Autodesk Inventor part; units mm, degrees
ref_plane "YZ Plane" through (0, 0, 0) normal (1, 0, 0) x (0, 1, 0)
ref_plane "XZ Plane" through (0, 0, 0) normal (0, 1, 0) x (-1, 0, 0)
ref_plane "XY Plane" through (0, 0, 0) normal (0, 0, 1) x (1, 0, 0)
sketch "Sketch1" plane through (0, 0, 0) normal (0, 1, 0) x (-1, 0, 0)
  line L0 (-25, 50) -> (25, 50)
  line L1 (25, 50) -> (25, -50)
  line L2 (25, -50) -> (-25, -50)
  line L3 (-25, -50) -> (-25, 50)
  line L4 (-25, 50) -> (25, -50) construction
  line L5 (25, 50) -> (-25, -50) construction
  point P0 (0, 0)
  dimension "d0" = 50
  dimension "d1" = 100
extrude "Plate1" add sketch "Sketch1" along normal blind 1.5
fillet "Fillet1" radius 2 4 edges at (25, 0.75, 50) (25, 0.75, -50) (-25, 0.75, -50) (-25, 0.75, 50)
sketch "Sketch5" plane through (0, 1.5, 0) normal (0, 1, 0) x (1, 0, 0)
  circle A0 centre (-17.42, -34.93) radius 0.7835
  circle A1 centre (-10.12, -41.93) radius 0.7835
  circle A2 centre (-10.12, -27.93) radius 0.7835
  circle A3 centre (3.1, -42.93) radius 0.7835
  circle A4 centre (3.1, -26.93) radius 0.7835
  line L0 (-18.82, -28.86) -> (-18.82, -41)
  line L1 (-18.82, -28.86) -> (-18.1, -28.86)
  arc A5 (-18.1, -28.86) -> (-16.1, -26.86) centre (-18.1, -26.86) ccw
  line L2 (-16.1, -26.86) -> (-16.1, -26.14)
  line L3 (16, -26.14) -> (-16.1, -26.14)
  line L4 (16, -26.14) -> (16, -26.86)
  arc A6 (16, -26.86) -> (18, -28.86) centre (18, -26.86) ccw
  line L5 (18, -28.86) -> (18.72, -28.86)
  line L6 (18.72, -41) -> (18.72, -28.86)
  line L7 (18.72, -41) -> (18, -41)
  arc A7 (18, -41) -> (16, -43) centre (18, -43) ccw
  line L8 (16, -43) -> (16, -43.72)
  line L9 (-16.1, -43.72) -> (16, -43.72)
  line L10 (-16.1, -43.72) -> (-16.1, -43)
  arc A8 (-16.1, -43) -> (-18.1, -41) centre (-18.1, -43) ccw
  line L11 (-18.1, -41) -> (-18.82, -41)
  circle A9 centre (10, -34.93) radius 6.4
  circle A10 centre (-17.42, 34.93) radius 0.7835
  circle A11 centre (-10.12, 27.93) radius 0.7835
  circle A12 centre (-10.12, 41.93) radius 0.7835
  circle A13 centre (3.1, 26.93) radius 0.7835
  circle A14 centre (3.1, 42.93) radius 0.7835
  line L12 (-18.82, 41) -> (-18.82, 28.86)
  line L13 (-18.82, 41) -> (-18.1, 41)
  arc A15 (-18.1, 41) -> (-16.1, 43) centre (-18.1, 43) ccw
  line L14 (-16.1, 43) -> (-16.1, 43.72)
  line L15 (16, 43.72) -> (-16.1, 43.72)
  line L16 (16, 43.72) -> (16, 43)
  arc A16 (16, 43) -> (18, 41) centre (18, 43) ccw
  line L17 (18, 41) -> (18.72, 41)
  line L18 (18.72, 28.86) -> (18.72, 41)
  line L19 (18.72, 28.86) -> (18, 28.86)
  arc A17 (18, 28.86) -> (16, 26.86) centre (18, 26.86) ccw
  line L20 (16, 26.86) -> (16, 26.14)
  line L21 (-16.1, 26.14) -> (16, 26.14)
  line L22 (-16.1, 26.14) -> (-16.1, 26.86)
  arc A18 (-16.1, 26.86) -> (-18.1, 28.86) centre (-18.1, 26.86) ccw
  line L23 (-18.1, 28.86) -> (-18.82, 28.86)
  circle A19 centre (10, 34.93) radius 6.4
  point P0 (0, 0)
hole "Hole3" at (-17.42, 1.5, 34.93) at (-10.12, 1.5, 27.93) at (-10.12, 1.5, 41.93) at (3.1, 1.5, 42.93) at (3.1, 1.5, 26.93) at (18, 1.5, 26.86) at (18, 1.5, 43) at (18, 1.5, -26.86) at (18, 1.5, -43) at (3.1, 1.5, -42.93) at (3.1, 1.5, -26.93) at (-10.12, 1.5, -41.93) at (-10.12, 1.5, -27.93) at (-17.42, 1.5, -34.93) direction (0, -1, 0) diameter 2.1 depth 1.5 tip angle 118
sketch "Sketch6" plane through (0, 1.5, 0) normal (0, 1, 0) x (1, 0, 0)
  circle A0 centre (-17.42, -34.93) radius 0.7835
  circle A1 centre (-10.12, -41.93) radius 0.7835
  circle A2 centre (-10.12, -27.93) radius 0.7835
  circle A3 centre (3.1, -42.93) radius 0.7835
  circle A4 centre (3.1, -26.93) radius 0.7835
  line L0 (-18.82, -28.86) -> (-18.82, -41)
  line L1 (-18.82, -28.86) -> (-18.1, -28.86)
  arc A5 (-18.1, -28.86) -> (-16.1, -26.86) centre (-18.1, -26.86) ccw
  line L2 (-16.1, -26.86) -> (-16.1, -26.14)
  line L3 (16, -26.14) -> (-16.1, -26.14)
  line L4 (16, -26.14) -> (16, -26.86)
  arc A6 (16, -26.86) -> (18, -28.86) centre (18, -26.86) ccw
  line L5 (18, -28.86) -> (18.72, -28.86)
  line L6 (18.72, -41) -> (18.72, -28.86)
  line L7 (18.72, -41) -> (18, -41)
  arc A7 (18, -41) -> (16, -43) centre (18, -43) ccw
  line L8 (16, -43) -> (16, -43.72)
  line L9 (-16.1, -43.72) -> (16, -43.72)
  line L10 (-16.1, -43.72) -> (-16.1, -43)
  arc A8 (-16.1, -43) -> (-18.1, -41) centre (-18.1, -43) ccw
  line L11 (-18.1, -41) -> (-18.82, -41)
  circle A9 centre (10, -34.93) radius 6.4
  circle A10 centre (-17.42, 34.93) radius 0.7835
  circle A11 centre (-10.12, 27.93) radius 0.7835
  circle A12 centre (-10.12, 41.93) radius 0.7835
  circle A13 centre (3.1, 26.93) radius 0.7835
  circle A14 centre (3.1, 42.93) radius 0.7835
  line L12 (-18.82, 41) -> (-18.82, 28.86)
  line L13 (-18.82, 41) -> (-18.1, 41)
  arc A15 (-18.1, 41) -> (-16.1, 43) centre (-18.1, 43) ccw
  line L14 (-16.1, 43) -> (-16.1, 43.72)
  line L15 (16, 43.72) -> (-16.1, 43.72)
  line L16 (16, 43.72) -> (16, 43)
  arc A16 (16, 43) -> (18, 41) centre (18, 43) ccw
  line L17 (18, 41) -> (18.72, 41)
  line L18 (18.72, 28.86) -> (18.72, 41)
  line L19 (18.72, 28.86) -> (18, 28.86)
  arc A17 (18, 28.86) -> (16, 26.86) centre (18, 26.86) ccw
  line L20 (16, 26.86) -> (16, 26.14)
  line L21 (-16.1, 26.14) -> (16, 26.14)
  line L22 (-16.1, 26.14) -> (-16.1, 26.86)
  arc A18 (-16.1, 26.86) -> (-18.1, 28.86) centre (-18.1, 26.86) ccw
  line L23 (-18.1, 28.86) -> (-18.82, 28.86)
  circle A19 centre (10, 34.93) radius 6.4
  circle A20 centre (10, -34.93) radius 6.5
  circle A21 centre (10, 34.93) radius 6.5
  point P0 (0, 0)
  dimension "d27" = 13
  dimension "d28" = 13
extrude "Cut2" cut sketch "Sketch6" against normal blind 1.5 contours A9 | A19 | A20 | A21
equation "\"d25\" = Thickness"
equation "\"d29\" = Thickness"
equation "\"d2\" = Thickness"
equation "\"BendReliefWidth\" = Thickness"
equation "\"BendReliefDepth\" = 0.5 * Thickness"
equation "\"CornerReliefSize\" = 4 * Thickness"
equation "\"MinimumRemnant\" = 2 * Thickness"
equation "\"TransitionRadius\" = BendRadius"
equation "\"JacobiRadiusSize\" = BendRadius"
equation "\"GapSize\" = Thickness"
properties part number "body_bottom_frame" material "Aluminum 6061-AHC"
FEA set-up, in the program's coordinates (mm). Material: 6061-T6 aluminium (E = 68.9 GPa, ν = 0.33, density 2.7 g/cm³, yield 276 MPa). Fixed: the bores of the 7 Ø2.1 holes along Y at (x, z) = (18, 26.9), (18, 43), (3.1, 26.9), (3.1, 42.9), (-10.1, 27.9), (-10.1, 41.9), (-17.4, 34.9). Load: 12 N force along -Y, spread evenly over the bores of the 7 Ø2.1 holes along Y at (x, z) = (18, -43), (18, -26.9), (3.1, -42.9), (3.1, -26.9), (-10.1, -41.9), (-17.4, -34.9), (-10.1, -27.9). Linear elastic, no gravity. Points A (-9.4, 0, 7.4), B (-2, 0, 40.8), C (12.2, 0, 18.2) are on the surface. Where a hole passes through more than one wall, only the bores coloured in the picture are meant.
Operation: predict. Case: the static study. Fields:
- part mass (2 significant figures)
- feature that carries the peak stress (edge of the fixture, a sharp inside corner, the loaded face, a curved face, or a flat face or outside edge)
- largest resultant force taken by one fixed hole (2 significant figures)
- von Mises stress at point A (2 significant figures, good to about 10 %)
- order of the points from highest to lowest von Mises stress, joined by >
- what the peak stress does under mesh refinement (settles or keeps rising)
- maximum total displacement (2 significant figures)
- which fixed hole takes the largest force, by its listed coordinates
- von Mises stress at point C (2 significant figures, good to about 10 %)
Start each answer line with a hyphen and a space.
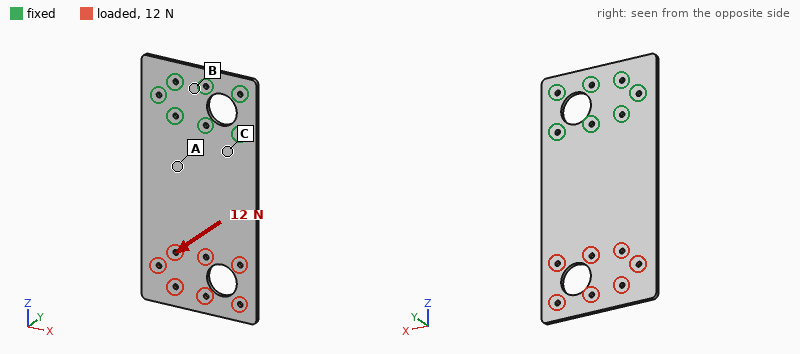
- 19 g
- edge of the fixture
- 19 N
- 24 MPa
- C > A > B
- keeps rising
- 1.3 mm
- (-10.1, 27.9)
- 32 MPa
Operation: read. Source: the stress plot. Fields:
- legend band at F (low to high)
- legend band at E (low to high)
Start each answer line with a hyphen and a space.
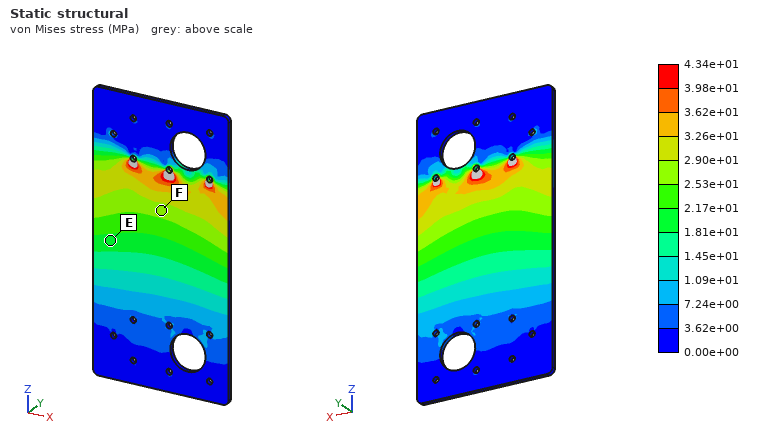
- 2.53e+01 to 2.90e+01 MPa
- 1.81e+01 to 2.17e+01 MPa
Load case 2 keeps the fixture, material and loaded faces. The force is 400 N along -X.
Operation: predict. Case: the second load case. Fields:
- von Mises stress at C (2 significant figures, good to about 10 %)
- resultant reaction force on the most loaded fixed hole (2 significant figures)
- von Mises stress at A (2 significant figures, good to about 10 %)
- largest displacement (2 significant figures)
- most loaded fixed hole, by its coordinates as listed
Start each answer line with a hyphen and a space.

- 23 MPa
- 600 N
- 15 MPa
- 74 µm
- (18, 26.9)
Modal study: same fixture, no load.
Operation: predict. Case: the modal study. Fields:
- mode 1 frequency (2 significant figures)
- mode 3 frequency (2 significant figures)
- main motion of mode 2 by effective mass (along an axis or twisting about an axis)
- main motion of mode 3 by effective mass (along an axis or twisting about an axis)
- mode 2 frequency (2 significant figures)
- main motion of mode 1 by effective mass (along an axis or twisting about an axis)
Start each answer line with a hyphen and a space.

- 220 Hz
- 1300 Hz
- twisting about Z
- along Y
- 700 Hz
- along Y
